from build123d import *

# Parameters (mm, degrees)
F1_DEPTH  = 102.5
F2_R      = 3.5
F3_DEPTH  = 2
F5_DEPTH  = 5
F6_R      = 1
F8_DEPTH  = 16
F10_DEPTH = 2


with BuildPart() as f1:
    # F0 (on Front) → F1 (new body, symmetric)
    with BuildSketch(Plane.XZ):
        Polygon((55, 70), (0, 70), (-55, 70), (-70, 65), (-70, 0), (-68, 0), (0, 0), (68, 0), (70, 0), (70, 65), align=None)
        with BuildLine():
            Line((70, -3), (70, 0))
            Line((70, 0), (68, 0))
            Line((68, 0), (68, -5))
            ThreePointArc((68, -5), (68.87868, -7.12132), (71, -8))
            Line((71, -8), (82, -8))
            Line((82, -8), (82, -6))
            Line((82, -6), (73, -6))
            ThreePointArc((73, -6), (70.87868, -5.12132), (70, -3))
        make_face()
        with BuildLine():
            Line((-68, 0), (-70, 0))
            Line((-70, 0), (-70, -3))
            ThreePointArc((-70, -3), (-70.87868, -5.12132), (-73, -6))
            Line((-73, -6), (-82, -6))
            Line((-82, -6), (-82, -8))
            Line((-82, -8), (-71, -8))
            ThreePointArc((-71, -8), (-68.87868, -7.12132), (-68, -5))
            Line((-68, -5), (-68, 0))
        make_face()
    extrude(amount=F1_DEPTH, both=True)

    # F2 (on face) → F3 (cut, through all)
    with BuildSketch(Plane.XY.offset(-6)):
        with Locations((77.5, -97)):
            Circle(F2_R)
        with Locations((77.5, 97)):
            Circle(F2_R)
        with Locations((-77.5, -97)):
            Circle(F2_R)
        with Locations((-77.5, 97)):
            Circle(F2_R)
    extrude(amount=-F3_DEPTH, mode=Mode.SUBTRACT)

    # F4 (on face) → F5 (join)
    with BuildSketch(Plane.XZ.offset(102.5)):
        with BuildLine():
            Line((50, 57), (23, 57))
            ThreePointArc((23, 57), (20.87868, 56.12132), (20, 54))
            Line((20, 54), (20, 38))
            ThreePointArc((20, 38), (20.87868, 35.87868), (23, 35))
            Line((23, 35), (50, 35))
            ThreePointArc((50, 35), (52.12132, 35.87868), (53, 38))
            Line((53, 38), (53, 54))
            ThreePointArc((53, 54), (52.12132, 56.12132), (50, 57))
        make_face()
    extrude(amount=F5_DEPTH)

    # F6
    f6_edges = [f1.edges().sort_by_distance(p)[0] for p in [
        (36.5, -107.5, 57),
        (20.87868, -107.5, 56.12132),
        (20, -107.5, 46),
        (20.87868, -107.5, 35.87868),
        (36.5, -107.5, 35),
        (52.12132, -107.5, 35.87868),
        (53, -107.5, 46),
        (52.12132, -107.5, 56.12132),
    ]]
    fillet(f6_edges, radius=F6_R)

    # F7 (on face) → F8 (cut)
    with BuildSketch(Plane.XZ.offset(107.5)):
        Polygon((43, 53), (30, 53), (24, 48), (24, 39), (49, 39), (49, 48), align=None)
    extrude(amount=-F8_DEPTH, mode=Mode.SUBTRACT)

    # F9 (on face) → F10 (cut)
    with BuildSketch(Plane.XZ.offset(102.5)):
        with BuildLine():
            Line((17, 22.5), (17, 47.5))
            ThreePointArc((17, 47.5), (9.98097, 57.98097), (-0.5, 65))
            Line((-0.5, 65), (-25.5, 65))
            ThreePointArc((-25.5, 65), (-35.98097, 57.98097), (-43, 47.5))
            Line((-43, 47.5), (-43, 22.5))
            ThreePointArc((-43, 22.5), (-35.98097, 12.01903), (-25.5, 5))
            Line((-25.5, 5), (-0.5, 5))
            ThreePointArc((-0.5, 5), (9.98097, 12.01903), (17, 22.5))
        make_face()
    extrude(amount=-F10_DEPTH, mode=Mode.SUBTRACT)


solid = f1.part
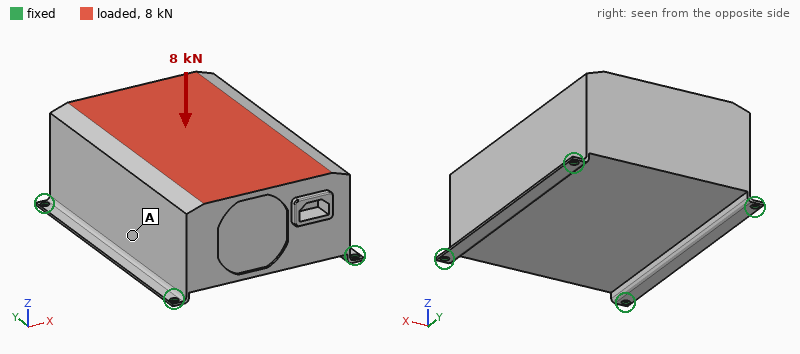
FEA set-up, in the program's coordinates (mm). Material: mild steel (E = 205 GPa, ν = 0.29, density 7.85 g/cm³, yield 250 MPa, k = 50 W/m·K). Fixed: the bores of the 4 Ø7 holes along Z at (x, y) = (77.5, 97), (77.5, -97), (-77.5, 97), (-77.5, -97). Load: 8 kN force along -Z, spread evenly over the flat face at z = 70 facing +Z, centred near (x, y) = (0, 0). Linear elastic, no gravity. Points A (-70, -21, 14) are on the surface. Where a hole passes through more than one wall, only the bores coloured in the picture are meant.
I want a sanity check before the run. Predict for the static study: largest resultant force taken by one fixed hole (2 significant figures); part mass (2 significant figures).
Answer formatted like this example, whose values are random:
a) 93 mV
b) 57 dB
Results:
a) 2.4 kN
b) 16 kg
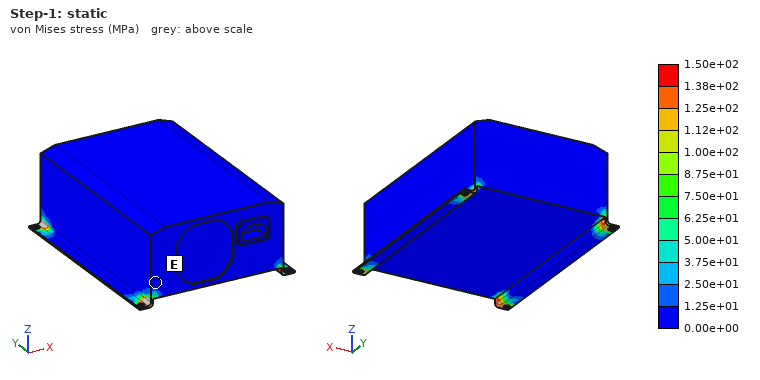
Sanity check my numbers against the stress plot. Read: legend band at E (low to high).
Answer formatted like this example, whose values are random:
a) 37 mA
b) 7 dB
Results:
a) 0.00e+00 to 1.25e+01 MPa
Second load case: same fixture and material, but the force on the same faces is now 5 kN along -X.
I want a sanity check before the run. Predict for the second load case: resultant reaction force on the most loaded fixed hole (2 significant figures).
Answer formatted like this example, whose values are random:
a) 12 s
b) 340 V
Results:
a) 1.9 kN
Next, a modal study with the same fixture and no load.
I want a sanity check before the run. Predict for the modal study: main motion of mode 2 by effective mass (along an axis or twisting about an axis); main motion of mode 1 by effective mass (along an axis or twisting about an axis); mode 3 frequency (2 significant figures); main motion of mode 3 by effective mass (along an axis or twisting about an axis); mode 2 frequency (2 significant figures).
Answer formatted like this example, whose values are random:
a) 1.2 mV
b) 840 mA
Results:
a) along Z
b) along X
c) 930 Hz
d) along Y
e) 770 Hz
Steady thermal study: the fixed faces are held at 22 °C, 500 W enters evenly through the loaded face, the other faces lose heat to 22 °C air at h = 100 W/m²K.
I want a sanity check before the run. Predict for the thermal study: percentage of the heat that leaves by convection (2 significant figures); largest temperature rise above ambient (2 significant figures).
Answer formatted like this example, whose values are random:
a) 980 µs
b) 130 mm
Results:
a) 95 %
b) 73 K
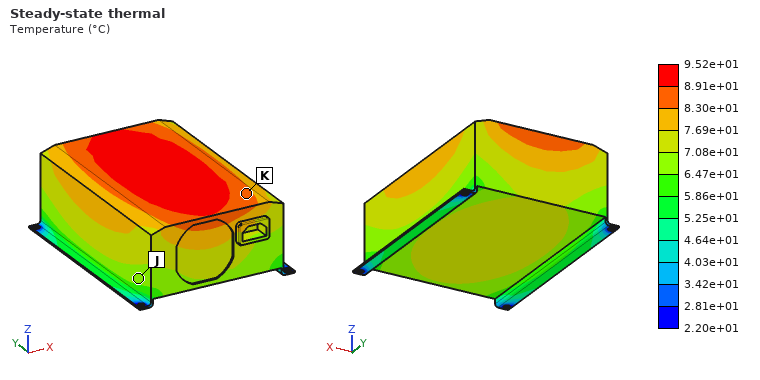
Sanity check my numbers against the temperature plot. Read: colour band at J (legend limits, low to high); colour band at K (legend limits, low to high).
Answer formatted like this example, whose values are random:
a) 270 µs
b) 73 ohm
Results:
a) 6.47e+01 to 7.08e+01 °C
b) 8.30e+01 to 8.91e+01 °C
